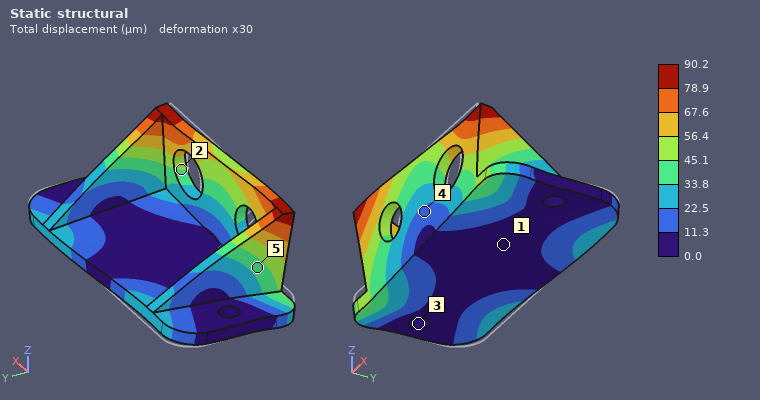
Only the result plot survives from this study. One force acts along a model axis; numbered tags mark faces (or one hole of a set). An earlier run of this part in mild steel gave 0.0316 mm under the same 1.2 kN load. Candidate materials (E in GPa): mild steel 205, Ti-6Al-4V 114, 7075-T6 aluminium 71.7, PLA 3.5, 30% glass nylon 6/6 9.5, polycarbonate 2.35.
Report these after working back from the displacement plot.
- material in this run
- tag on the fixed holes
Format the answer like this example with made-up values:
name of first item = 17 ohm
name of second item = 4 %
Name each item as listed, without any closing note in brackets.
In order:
material in this run = 7075-T6 aluminium
tag on the fixed holes = 3
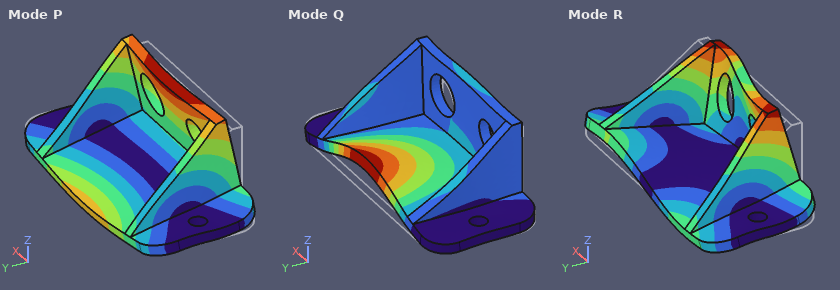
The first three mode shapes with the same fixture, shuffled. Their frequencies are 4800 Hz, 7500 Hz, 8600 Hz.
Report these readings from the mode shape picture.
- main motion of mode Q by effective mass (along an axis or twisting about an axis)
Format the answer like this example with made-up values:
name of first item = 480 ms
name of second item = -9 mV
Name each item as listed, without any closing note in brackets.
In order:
main motion of mode Q by effective mass = along Z
